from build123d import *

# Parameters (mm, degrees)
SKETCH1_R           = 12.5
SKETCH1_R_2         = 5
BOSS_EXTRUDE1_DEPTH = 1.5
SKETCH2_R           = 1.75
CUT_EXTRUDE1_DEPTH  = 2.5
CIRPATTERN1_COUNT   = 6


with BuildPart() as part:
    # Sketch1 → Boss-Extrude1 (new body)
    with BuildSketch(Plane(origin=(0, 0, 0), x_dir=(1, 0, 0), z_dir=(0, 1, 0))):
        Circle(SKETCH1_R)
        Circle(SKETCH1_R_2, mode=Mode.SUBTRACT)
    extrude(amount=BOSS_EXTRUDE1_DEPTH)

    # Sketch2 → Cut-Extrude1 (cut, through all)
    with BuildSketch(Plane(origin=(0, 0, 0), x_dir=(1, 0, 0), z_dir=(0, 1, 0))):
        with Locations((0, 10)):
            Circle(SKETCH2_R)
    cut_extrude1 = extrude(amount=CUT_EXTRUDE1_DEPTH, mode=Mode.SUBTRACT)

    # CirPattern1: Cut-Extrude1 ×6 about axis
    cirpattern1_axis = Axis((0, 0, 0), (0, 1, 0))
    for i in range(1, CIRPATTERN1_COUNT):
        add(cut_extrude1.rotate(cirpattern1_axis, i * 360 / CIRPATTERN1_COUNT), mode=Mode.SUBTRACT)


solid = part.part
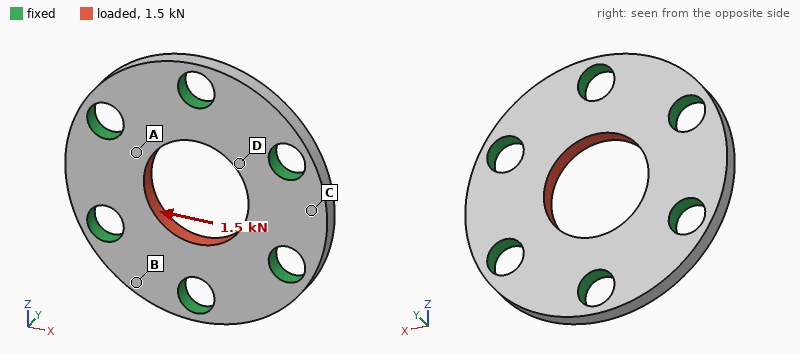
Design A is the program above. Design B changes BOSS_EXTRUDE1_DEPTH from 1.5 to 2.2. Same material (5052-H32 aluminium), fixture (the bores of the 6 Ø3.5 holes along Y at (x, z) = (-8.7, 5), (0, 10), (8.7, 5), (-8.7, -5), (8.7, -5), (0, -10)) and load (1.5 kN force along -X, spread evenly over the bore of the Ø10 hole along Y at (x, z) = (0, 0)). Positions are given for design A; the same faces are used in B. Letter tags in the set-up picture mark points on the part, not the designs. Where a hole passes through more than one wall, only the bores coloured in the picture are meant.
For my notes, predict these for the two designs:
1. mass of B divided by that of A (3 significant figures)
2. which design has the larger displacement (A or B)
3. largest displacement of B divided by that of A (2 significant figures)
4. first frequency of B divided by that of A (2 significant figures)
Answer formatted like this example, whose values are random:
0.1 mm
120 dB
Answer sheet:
1.47
A
0.68
1.3
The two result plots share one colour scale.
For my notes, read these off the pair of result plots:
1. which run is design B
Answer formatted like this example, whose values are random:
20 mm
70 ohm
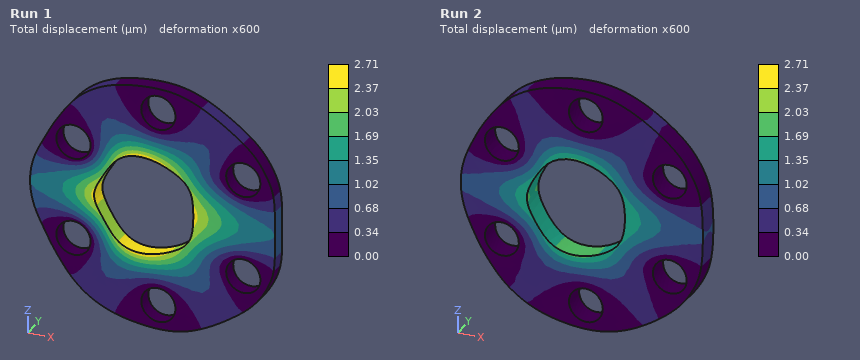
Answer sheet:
Run 2
